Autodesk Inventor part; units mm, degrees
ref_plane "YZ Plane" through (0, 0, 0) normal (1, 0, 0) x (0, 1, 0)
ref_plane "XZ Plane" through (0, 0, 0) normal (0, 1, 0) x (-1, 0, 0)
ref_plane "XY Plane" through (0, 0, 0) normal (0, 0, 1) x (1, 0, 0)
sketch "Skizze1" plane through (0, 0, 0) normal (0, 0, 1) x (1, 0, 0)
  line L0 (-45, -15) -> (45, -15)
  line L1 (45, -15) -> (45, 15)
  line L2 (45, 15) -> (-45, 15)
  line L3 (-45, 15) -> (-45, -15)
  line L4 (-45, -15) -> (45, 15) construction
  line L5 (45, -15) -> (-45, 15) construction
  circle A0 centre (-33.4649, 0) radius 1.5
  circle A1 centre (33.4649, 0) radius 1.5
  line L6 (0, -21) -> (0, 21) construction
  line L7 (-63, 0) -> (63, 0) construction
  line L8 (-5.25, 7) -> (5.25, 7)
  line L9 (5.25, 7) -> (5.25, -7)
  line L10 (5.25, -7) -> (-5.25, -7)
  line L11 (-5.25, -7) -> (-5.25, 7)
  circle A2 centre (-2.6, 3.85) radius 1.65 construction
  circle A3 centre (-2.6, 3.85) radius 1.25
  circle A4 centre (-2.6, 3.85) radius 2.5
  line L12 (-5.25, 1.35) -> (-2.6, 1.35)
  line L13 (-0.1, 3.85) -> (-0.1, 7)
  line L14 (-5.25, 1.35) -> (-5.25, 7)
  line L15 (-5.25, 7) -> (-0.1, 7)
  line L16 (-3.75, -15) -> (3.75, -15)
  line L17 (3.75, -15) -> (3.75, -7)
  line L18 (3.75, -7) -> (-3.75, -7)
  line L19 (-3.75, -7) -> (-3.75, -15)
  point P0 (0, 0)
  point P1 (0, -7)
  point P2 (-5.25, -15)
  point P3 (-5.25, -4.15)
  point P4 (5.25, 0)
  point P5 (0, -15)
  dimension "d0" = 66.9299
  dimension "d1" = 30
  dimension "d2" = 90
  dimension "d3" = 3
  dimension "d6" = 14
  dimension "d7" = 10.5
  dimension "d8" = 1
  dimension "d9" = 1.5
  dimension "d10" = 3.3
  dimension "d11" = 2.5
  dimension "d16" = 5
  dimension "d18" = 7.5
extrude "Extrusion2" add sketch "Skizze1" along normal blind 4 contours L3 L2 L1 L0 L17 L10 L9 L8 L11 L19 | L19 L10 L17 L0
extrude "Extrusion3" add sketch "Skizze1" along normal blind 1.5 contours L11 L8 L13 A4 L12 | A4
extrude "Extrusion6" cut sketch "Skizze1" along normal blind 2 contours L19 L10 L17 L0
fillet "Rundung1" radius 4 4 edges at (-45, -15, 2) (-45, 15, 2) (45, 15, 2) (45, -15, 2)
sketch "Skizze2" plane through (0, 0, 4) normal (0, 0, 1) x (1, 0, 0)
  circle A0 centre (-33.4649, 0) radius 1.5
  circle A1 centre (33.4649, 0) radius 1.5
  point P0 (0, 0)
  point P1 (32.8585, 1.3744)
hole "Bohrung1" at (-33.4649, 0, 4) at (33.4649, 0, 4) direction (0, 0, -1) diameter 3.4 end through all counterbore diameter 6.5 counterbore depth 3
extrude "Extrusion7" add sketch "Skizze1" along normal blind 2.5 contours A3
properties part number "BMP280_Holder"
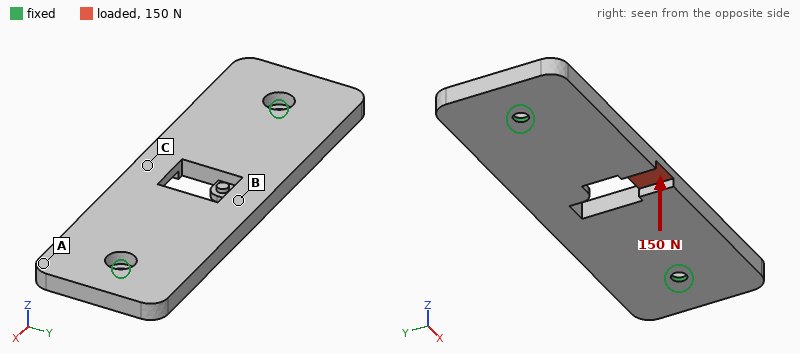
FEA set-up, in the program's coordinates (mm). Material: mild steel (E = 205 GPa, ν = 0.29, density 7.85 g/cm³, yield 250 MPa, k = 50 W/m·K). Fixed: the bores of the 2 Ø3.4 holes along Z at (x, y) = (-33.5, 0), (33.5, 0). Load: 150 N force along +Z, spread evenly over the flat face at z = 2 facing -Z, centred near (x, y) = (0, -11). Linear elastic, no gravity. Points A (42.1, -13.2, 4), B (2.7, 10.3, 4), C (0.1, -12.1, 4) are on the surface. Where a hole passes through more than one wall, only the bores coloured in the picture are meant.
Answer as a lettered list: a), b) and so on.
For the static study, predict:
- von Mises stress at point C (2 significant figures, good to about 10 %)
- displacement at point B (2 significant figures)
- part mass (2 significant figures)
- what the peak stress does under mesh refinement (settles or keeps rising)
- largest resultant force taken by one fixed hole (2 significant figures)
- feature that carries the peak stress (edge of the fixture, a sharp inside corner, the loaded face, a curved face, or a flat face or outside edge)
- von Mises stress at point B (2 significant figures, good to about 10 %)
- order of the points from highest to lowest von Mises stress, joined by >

a) 66 MPa
b) 9.3 µm
c) 77 g
d) keeps rising
e) 460 N
f) edge of the fixture
g) 33 MPa
h) C > B > A
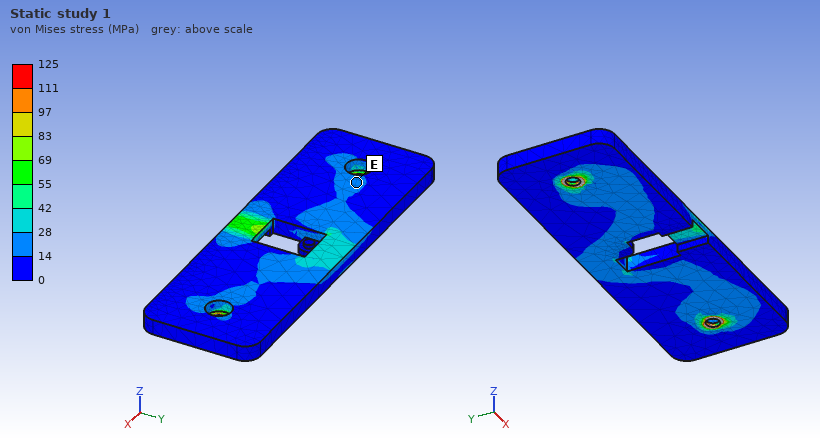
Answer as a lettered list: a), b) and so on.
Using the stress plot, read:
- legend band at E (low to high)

a) 14 to 28 MPa
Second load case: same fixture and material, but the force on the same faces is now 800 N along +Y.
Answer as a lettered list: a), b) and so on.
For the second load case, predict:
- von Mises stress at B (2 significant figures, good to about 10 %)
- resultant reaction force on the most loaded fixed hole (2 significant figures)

a) 21 MPa
b) 410 N
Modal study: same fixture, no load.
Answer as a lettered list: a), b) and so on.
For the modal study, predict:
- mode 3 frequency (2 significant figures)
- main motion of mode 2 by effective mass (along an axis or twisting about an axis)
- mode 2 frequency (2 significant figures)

a) 5000 Hz
b) along Z
c) 2700 Hz
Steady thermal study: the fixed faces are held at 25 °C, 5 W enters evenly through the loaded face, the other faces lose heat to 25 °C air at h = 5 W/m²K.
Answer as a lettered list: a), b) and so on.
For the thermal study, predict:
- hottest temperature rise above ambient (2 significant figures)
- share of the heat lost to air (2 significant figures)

a) 37 K
b) 7.2 %
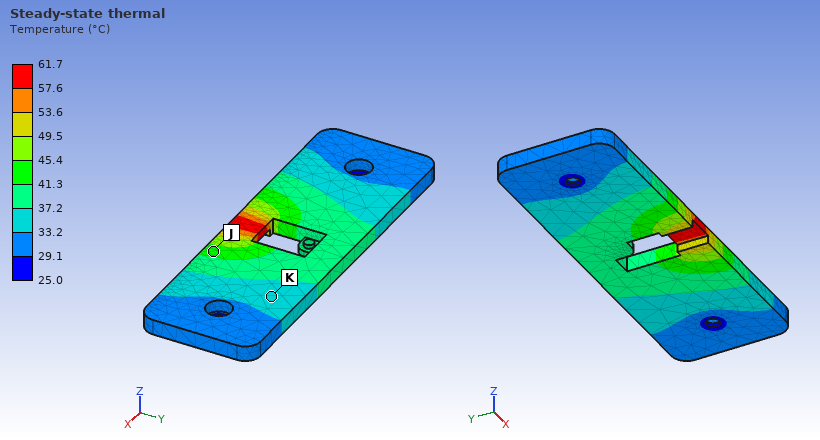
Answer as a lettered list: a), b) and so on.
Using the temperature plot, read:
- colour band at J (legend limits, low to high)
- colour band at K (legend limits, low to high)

a) 41.3 to 45.4 °C
b) 33.2 to 37.2 °C
